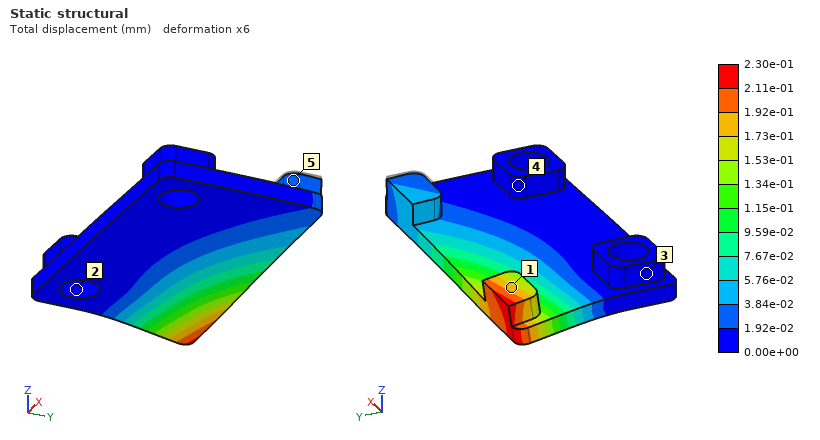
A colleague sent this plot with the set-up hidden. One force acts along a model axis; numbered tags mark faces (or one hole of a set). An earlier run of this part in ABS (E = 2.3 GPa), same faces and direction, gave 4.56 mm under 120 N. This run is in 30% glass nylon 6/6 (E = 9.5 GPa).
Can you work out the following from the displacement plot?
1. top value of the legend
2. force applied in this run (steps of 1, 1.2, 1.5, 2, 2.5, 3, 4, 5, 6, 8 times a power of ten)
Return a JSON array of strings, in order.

["2.30e-01 mm", "25 N"]
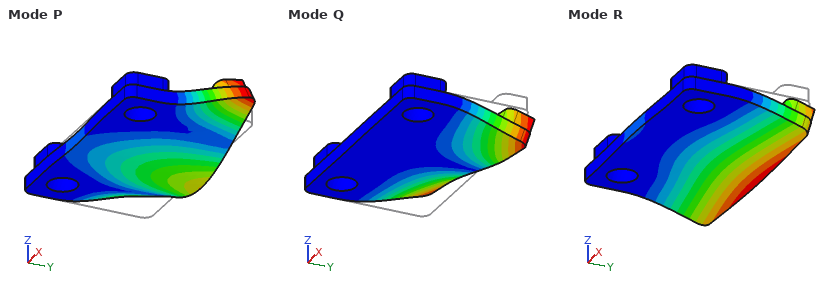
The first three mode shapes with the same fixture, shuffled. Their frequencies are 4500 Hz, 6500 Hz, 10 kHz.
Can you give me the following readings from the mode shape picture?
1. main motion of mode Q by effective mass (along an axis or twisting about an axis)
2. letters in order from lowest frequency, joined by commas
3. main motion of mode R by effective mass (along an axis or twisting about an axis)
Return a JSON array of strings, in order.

["twisting about Y", "R, Q, P", "along Z"]
